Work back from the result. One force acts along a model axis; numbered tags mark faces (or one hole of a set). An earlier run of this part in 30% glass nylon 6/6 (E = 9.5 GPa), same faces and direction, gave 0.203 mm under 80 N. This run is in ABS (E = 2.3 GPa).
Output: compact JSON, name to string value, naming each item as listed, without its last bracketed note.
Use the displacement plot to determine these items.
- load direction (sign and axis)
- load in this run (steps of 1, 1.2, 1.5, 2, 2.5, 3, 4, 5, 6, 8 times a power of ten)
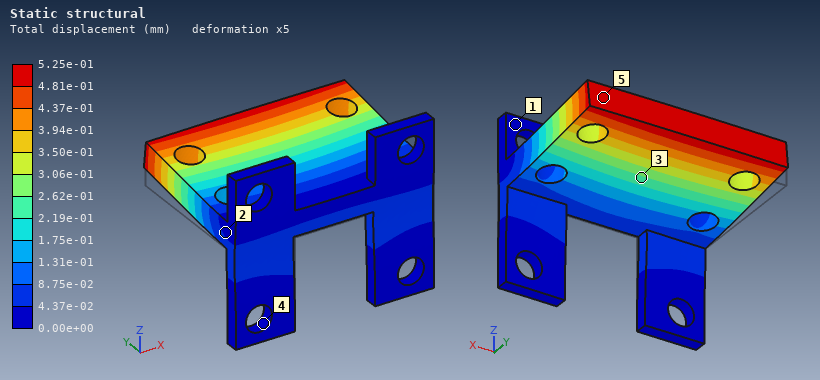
{"load direction": "+Z", "load in this run": "50 N"}
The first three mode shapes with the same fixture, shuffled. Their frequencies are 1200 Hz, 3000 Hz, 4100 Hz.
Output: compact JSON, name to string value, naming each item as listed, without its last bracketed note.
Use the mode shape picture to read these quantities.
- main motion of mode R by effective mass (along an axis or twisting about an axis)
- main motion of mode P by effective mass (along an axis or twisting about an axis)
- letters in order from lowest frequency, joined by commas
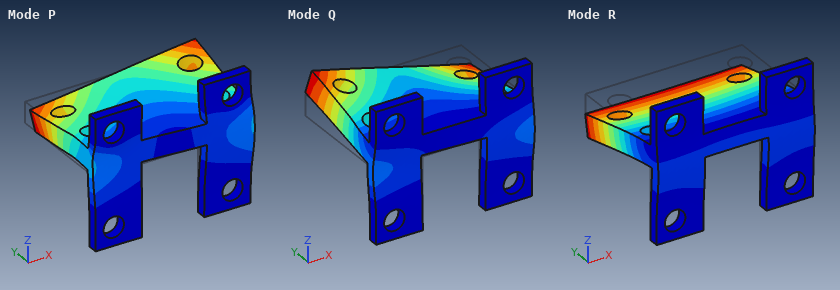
{"main motion of mode R by effective mass": "along Z", "main motion of mode P by effective mass": "along X", "letters in order from lowest frequency, joined by commas": "R, Q, P"}
